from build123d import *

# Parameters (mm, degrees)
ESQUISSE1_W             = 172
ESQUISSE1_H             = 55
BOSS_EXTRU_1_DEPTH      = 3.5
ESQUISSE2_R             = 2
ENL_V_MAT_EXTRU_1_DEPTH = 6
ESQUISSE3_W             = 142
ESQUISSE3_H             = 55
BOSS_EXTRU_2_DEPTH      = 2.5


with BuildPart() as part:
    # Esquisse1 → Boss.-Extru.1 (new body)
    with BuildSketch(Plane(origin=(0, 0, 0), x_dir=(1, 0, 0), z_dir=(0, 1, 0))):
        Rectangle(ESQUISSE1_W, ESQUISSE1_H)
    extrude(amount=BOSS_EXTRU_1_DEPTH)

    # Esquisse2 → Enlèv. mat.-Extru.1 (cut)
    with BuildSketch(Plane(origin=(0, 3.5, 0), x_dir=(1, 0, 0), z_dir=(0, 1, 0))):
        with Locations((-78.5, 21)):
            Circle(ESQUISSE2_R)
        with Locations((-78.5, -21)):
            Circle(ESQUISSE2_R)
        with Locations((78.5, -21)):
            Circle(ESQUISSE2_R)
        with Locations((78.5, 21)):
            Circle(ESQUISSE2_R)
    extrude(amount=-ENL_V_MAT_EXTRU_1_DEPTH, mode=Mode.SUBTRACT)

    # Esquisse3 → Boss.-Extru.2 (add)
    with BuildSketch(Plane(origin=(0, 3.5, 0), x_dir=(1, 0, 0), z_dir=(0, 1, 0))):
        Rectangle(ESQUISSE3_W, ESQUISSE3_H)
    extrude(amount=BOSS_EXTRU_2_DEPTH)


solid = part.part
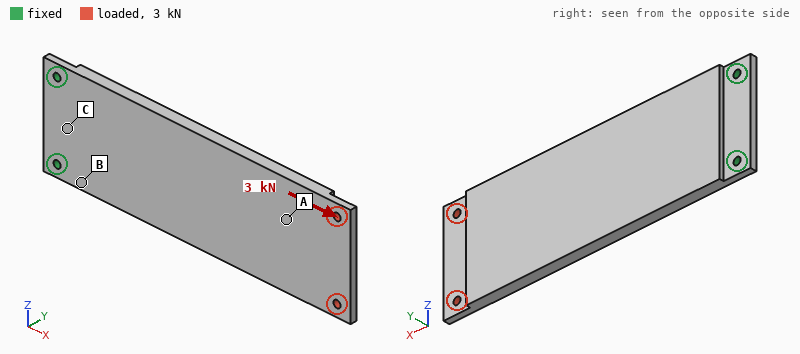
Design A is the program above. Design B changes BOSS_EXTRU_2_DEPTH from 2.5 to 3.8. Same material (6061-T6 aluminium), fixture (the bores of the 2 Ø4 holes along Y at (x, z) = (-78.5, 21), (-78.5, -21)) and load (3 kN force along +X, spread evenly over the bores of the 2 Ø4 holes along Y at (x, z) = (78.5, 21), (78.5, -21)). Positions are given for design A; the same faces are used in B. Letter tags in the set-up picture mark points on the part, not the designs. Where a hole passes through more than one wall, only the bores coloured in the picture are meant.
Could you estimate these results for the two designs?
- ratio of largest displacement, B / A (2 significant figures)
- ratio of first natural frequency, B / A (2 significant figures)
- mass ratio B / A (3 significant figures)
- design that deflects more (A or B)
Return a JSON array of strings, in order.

["0.85", "1.0", "1.19", "A"]
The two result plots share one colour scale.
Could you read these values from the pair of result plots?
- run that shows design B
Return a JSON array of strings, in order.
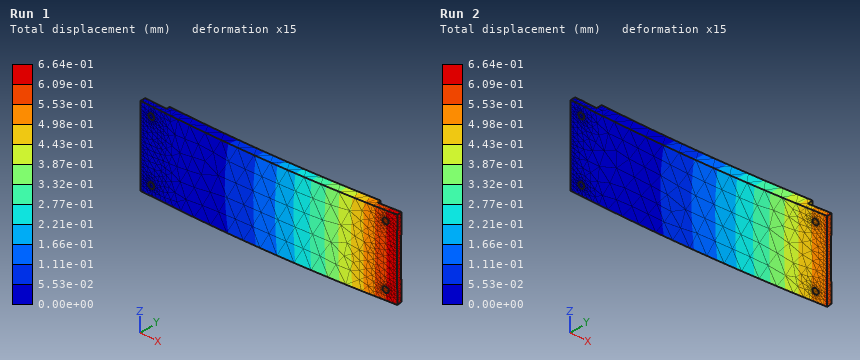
["Run 2"]
